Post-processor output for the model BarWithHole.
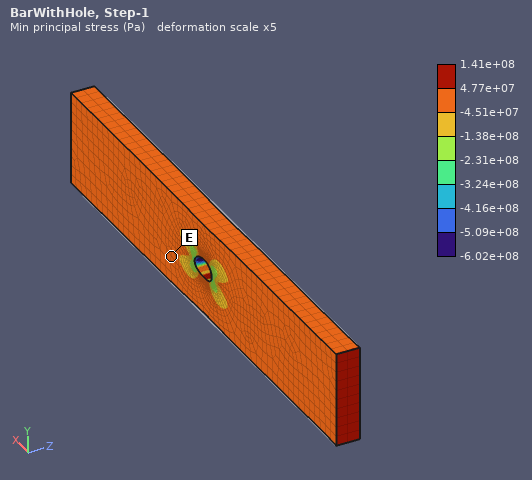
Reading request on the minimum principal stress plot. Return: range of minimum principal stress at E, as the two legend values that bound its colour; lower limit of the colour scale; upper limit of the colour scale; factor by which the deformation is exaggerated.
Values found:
-4.51e+07 to 4.77e+07 Pa
-6.02e+08 Pa
1.41e+08 Pa
5
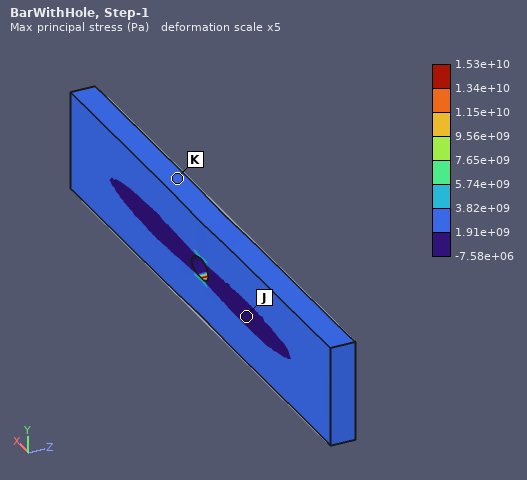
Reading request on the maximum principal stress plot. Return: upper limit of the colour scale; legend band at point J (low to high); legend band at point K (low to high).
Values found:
1.53e+10 Pa
-7.58e+06 to 1.91e+09 Pa
1.91e+09 to 3.82e+09 Pa
